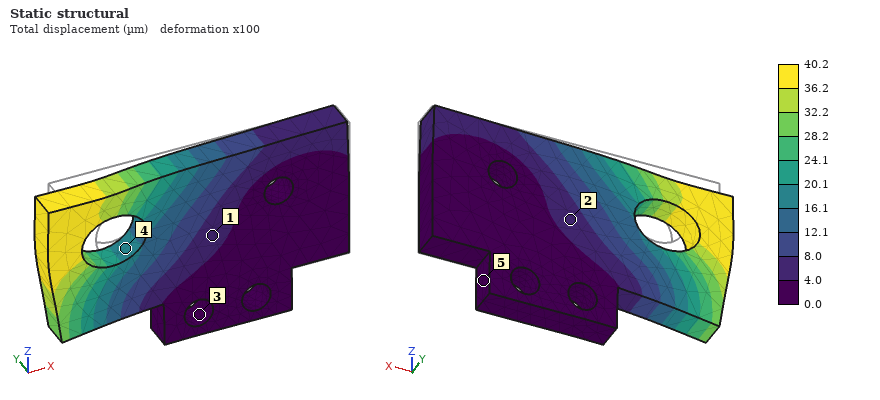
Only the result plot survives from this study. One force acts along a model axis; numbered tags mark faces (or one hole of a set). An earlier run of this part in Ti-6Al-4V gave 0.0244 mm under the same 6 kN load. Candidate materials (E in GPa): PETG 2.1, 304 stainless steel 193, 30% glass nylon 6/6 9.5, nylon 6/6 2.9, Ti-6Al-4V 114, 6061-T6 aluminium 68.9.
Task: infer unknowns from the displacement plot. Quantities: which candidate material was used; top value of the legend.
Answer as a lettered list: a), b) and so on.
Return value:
a) 6061-T6 aluminium
b) 40.2 µm
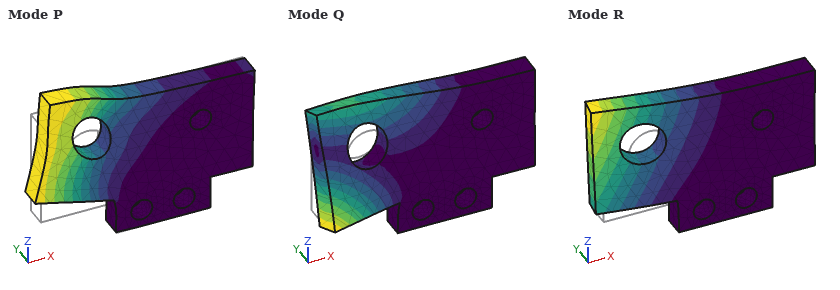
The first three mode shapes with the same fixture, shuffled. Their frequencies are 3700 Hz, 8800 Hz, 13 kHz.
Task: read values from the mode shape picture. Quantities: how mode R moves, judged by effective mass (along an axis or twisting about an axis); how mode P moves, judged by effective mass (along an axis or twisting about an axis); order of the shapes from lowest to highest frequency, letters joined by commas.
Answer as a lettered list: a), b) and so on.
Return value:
a) along Y
b) along Z
c) R, Q, P
